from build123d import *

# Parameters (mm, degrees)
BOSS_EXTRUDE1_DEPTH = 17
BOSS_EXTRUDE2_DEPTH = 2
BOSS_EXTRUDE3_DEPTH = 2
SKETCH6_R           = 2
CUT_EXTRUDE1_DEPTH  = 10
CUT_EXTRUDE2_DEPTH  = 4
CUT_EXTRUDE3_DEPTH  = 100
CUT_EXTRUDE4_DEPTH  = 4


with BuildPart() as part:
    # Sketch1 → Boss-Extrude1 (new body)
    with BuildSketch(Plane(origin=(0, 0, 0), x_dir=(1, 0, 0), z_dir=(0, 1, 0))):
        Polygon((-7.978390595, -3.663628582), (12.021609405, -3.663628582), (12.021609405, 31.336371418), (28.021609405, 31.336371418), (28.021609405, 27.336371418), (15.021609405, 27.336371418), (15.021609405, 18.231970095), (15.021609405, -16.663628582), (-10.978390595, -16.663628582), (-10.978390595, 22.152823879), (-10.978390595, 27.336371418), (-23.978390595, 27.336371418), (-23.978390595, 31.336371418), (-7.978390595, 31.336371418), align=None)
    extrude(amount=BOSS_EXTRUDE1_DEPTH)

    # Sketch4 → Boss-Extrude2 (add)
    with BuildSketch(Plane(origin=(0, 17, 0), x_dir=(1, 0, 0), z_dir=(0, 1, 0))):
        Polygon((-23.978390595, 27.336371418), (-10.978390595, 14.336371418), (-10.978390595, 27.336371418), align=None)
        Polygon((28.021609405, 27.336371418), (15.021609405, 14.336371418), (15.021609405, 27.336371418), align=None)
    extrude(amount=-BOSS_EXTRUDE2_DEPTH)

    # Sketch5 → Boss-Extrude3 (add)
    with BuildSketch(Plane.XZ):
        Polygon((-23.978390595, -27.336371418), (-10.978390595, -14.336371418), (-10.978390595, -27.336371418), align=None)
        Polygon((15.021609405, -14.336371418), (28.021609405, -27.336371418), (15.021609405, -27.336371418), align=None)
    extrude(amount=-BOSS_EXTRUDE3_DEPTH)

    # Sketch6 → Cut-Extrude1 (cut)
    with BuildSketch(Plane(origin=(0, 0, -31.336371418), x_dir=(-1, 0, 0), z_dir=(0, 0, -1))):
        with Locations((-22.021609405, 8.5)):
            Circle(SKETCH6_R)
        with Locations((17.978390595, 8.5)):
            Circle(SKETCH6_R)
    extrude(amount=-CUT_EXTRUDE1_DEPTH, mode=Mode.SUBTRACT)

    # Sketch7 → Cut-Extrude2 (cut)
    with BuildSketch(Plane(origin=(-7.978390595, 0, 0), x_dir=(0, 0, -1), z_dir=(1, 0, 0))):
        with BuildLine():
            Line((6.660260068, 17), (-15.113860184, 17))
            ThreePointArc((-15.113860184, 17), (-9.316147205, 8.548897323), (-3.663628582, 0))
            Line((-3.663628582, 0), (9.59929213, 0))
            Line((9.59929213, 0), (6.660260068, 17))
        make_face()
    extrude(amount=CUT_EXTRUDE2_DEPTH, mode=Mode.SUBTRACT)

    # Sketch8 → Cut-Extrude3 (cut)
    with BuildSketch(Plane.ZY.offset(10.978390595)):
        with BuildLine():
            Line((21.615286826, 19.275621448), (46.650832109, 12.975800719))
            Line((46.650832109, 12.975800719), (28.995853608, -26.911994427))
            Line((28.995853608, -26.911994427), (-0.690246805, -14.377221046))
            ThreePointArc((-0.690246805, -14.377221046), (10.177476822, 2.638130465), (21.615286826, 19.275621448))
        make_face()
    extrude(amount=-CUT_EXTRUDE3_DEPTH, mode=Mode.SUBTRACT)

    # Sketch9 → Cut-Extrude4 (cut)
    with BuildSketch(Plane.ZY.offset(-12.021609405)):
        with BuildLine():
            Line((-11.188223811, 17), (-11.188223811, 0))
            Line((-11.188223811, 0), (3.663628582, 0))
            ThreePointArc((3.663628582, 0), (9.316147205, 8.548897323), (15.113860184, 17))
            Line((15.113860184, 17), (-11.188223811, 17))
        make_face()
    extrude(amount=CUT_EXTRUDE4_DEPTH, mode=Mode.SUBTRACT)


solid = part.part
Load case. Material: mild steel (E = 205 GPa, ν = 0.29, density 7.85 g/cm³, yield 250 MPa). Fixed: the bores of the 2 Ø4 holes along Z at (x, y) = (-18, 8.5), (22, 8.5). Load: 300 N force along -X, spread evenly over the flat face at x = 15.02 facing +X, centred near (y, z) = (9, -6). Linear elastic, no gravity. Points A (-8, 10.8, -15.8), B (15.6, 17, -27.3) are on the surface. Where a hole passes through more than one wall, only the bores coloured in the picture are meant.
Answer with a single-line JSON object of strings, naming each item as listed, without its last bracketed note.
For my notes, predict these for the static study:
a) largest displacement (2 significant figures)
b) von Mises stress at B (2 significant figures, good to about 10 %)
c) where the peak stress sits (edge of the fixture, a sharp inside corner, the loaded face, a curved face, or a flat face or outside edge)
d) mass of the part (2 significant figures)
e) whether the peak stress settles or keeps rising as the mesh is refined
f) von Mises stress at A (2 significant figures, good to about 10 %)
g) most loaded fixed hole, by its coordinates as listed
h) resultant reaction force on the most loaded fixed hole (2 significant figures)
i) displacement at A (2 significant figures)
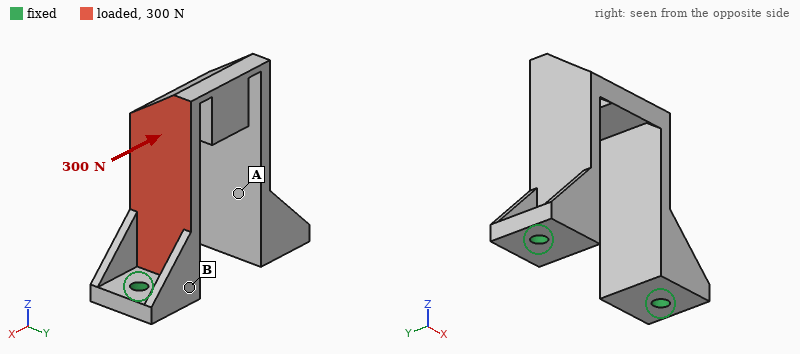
{"largest displacement": "29 µm", "von Mises stress at B": "11 MPa", "where the peak stress sits": "edge of the fixture", "mass of the part": "75 g", "whether the peak stress settles or keeps rising as the mesh is refined": "keeps rising", "von Mises stress at A": "21 MPa", "most loaded fixed hole, by its coordinates as listed": "(22, 8.5)", "resultant reaction force on the most loaded fixed hole": "230 N", "displacement at A": "5.2 µm"}
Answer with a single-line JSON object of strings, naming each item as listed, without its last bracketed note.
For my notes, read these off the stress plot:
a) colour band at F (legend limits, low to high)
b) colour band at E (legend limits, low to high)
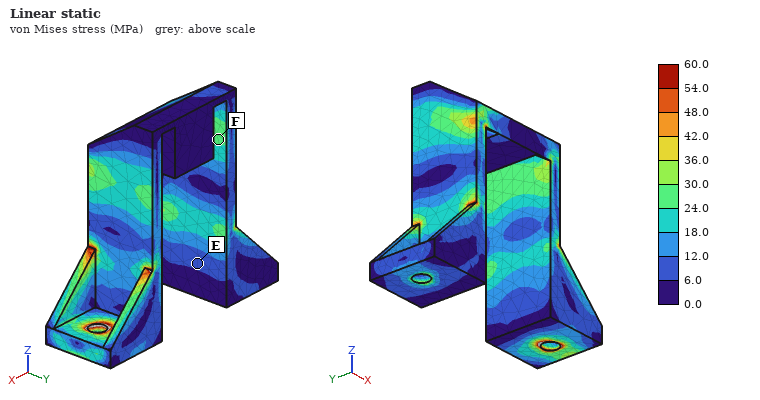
{"colour band at F": "24.0 to 30.0 MPa", "colour band at E": "6.0 to 12.0 MPa"}
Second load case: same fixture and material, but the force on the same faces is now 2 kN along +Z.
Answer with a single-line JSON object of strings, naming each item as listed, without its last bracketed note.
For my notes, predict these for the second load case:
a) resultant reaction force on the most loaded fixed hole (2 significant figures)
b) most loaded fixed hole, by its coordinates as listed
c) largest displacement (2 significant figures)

{"resultant reaction force on the most loaded fixed hole": "2.0 kN", "most loaded fixed hole, by its coordinates as listed": "(22, 8.5)", "largest displacement": "33 µm"}
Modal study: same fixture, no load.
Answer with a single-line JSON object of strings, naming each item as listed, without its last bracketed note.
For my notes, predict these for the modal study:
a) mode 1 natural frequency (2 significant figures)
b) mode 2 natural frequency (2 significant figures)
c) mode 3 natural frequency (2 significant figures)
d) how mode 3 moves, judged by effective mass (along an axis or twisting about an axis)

{"mode 1 natural frequency": "2100 Hz", "mode 2 natural frequency": "2100 Hz", "mode 3 natural frequency": "4200 Hz", "how mode 3 moves, judged by effective mass": "twisting about Z"}
